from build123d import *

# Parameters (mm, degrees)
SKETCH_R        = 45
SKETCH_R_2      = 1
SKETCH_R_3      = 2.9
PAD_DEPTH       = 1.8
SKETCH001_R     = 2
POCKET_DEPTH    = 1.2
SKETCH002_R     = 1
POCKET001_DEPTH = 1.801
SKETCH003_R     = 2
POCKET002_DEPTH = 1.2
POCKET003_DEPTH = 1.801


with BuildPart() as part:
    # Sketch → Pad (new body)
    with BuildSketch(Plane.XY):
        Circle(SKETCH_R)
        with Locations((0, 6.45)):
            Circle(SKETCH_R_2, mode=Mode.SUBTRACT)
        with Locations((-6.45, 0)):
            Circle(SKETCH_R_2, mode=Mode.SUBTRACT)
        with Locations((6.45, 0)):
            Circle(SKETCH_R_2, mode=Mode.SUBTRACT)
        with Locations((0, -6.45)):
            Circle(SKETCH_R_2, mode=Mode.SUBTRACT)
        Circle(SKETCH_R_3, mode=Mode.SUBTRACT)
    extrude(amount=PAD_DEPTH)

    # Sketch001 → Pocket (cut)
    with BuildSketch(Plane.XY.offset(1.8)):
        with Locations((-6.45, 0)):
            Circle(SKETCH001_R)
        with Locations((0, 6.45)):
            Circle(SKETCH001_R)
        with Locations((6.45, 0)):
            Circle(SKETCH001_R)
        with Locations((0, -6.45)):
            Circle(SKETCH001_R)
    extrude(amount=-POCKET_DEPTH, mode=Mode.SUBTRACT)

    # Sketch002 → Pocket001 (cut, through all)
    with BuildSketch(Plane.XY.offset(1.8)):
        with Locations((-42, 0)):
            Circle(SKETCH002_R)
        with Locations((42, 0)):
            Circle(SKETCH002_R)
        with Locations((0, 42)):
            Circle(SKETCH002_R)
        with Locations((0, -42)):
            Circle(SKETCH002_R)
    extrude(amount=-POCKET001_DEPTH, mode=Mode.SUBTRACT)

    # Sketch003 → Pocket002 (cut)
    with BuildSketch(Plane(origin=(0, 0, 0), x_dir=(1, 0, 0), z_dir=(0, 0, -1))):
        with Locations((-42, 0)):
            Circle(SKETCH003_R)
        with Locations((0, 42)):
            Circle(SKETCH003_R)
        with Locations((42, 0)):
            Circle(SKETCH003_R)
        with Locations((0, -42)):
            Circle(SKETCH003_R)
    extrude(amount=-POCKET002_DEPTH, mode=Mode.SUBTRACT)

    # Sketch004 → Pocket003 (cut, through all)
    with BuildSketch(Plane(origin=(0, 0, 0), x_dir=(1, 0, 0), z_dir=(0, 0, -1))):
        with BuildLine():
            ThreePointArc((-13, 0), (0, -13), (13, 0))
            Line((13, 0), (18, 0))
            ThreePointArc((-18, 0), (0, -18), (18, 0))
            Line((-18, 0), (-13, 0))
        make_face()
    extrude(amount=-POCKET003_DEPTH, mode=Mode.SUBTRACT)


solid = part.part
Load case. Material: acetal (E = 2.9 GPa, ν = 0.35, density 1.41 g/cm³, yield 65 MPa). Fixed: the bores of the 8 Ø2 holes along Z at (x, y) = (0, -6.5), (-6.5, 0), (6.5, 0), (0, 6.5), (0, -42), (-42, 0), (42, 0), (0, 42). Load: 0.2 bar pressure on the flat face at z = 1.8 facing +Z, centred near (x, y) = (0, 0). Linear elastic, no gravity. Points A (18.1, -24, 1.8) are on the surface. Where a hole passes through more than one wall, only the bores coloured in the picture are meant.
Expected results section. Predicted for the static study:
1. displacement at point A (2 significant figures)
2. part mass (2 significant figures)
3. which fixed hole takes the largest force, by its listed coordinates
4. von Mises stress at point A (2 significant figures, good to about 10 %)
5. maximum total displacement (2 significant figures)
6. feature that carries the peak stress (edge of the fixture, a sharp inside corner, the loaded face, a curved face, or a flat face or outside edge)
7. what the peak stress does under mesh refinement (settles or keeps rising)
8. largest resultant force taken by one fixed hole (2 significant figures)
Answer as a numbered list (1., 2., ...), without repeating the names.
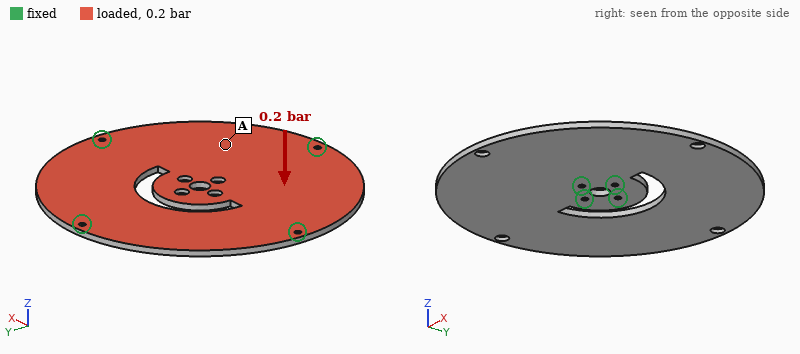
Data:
1. 0.42 mm
2. 15 g
3. (0, 42)
4. 2.6 MPa
5. 0.75 mm
6. edge of the fixture
7. keeps rising
8. 47 N
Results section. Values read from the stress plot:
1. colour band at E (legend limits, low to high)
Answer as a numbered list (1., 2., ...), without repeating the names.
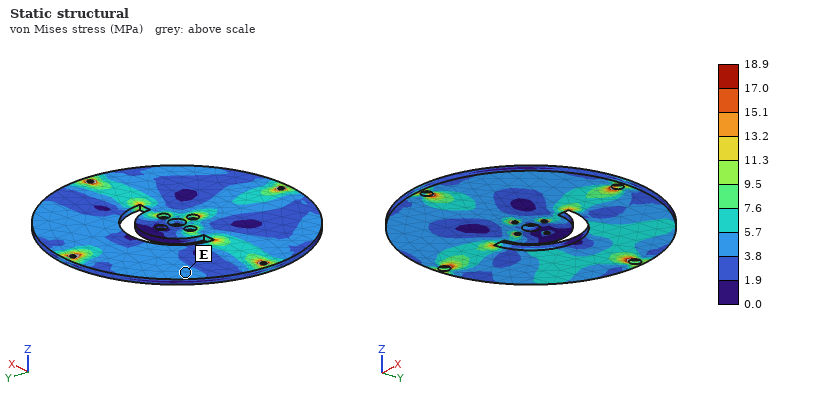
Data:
1. 3.8 to 5.7 MPa
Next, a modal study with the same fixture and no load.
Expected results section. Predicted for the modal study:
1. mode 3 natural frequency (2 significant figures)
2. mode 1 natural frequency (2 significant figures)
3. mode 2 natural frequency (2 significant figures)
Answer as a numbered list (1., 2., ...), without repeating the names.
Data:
1. 580 Hz
2. 470 Hz
3. 560 Hz
